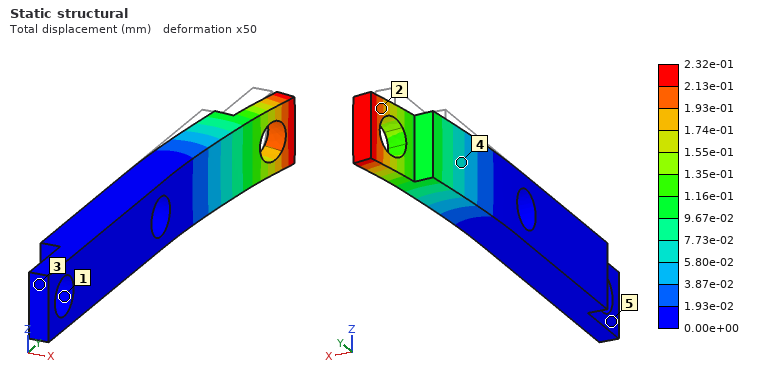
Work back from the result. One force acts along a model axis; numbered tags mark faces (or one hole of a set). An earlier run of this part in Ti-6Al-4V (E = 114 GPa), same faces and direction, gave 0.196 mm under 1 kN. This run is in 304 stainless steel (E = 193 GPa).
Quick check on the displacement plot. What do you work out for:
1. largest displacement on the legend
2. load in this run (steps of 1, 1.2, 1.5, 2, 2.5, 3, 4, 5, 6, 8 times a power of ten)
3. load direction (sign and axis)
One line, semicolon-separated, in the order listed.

2.32e-01 mm; 2 kN; +X
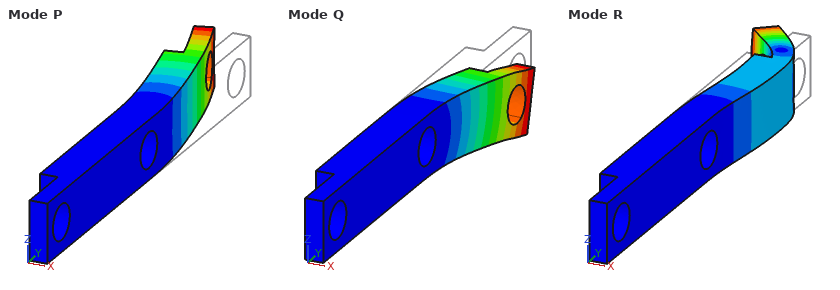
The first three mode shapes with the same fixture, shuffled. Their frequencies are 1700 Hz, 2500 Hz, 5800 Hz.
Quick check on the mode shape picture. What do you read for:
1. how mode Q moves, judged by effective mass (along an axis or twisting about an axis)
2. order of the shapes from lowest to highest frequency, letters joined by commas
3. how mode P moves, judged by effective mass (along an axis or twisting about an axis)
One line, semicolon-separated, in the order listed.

along Z; P, Q, R; along X
